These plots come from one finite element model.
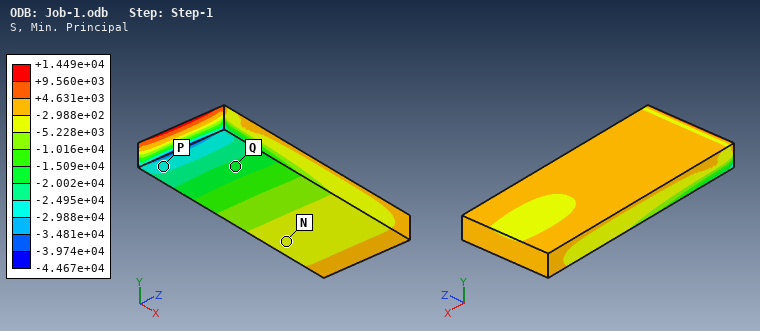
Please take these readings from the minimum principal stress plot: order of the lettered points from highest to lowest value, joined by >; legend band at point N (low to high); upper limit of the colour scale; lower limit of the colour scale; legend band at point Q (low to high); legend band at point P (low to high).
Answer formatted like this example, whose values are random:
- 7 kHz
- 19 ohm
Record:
- N > Q > P
- -5.228e+03 to -2.988e+02
- +1.449e+04
- -4.467e+04
- -2.002e+04 to -1.509e+04
- -2.988e+04 to -2.495e+04
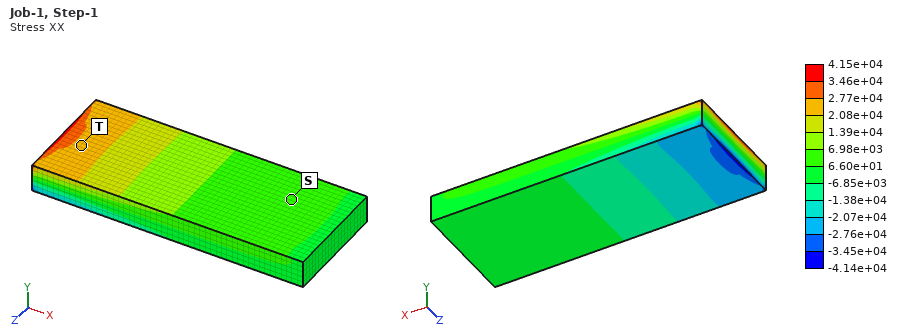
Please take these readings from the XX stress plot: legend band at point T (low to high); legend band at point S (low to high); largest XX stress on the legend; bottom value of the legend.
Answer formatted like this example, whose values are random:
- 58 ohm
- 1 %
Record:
- 2.08e+04 to 2.77e+04
- 6.60e+01 to 6.98e+03
- 4.15e+04
- -4.14e+04
